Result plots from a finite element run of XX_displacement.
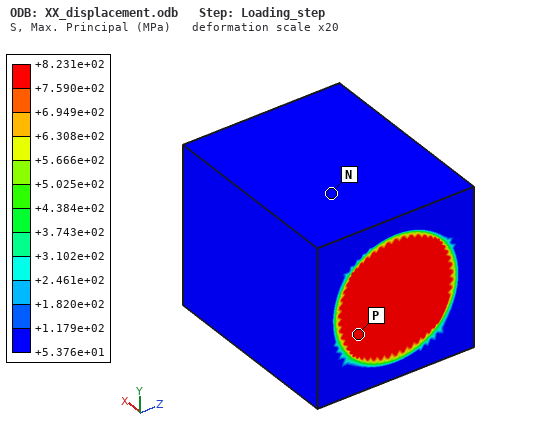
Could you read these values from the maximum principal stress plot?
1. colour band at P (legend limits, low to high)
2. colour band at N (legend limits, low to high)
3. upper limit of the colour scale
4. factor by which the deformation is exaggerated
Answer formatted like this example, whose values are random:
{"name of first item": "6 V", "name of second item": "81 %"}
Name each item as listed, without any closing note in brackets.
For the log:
{"colour band at P": "+7.590e+02 to +8.231e+02 MPa", "colour band at N": "+5.376e+01 to +1.179e+02 MPa", "upper limit of the colour scale": "+8.231e+02 MPa", "factor by which the deformation is exaggerated": "20"}
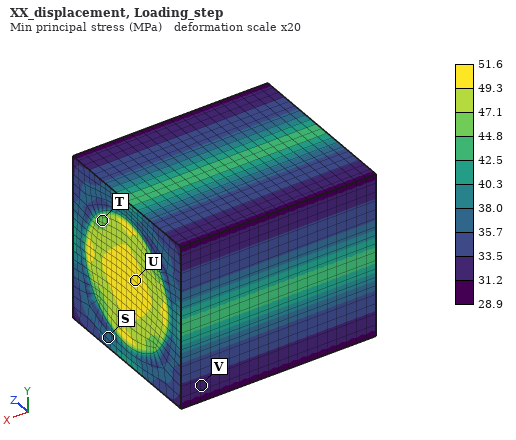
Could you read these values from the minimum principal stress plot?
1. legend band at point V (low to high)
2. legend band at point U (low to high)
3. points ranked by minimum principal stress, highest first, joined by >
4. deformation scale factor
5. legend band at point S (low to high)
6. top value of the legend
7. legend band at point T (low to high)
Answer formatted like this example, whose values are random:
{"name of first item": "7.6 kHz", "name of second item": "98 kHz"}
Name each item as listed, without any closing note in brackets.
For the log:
{"legend band at point V": "31.2 to 33.5 MPa", "legend band at point U": "49.3 to 51.6 MPa", "points ranked by minimum principal stress, highest first, joined by >": "U > T > S > V", "deformation scale factor": "20", "legend band at point S": "35.7 to 38.0 MPa", "top value of the legend": "51.6 MPa", "legend band at point T": "44.8 to 47.1 MPa"}
